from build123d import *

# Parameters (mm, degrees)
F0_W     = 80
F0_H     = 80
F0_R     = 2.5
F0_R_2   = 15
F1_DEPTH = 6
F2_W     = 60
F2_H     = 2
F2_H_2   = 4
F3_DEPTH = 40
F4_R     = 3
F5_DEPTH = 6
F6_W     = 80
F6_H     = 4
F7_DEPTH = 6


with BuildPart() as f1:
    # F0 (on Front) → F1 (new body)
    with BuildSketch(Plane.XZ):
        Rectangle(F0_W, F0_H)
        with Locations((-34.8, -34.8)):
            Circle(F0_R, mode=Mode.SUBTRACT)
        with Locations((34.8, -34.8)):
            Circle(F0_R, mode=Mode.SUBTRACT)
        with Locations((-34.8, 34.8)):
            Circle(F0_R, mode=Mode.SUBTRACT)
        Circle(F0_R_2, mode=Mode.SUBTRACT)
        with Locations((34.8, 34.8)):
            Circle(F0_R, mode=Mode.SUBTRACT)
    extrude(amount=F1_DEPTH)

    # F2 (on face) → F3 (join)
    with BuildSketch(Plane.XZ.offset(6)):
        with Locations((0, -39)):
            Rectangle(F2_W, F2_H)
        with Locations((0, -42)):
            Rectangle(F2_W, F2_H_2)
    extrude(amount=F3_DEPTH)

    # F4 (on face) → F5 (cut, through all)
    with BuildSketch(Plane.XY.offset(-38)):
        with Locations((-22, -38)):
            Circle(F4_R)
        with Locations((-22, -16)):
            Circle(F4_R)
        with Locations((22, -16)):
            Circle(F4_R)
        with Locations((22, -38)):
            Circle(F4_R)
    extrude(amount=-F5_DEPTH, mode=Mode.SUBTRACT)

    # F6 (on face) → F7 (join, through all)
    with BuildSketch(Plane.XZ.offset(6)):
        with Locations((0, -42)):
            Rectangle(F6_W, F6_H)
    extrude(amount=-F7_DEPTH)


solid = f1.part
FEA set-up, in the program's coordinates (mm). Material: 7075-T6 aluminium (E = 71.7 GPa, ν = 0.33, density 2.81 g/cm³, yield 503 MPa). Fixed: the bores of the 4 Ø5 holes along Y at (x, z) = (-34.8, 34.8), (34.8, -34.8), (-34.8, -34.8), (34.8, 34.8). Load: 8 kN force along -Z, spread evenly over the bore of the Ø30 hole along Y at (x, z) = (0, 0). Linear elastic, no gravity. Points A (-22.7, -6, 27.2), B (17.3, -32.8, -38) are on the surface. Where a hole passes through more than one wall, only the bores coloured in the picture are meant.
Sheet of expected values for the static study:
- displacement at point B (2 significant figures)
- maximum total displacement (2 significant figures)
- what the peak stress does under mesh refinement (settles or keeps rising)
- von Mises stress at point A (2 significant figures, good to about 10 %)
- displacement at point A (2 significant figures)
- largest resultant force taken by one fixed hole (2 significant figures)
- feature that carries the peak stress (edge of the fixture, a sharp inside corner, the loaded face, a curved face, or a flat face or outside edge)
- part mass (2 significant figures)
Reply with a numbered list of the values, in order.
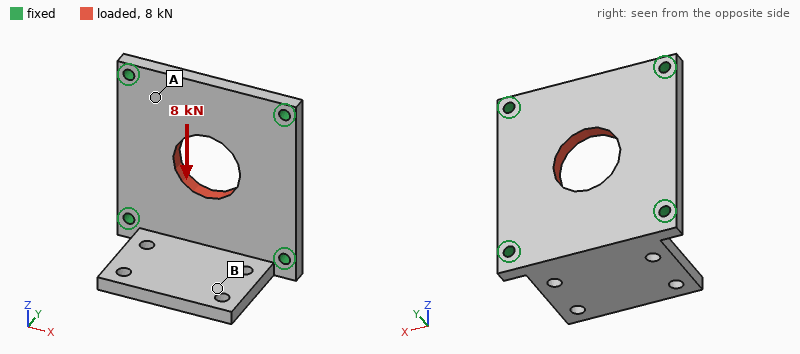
1. 9.4 µm
2. 15 µm
3. keeps rising
4. 17 MPa
5. 6.6 µm
6. 2.2 kN
7. edge of the fixture
8. 140 g
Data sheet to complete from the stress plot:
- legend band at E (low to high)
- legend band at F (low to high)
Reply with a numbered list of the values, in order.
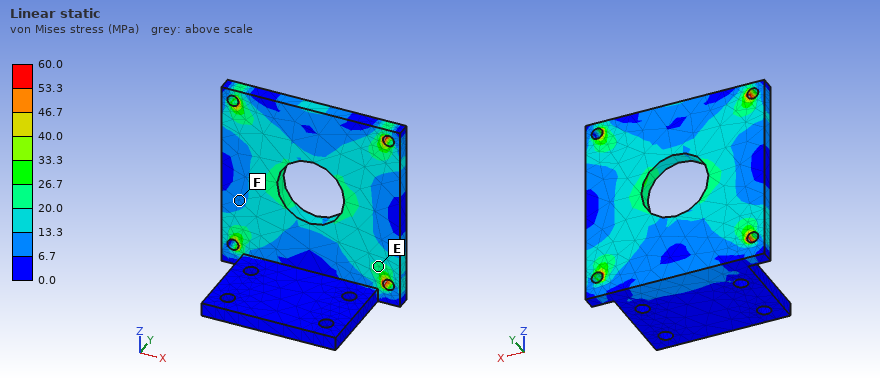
1. 20.0 to 26.7 MPa
2. 6.7 to 13.3 MPa
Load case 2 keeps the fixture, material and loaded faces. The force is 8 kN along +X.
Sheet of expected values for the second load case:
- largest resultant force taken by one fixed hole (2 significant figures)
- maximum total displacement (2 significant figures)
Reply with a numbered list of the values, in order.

1. 2.3 kN
2. 14 µm
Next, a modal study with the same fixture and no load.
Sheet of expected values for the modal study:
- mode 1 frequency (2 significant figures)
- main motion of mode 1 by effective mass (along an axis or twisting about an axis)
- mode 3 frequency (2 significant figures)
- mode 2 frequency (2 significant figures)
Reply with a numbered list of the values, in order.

1. 1900 Hz
2. along Z
3. 4700 Hz
4. 4600 Hz
